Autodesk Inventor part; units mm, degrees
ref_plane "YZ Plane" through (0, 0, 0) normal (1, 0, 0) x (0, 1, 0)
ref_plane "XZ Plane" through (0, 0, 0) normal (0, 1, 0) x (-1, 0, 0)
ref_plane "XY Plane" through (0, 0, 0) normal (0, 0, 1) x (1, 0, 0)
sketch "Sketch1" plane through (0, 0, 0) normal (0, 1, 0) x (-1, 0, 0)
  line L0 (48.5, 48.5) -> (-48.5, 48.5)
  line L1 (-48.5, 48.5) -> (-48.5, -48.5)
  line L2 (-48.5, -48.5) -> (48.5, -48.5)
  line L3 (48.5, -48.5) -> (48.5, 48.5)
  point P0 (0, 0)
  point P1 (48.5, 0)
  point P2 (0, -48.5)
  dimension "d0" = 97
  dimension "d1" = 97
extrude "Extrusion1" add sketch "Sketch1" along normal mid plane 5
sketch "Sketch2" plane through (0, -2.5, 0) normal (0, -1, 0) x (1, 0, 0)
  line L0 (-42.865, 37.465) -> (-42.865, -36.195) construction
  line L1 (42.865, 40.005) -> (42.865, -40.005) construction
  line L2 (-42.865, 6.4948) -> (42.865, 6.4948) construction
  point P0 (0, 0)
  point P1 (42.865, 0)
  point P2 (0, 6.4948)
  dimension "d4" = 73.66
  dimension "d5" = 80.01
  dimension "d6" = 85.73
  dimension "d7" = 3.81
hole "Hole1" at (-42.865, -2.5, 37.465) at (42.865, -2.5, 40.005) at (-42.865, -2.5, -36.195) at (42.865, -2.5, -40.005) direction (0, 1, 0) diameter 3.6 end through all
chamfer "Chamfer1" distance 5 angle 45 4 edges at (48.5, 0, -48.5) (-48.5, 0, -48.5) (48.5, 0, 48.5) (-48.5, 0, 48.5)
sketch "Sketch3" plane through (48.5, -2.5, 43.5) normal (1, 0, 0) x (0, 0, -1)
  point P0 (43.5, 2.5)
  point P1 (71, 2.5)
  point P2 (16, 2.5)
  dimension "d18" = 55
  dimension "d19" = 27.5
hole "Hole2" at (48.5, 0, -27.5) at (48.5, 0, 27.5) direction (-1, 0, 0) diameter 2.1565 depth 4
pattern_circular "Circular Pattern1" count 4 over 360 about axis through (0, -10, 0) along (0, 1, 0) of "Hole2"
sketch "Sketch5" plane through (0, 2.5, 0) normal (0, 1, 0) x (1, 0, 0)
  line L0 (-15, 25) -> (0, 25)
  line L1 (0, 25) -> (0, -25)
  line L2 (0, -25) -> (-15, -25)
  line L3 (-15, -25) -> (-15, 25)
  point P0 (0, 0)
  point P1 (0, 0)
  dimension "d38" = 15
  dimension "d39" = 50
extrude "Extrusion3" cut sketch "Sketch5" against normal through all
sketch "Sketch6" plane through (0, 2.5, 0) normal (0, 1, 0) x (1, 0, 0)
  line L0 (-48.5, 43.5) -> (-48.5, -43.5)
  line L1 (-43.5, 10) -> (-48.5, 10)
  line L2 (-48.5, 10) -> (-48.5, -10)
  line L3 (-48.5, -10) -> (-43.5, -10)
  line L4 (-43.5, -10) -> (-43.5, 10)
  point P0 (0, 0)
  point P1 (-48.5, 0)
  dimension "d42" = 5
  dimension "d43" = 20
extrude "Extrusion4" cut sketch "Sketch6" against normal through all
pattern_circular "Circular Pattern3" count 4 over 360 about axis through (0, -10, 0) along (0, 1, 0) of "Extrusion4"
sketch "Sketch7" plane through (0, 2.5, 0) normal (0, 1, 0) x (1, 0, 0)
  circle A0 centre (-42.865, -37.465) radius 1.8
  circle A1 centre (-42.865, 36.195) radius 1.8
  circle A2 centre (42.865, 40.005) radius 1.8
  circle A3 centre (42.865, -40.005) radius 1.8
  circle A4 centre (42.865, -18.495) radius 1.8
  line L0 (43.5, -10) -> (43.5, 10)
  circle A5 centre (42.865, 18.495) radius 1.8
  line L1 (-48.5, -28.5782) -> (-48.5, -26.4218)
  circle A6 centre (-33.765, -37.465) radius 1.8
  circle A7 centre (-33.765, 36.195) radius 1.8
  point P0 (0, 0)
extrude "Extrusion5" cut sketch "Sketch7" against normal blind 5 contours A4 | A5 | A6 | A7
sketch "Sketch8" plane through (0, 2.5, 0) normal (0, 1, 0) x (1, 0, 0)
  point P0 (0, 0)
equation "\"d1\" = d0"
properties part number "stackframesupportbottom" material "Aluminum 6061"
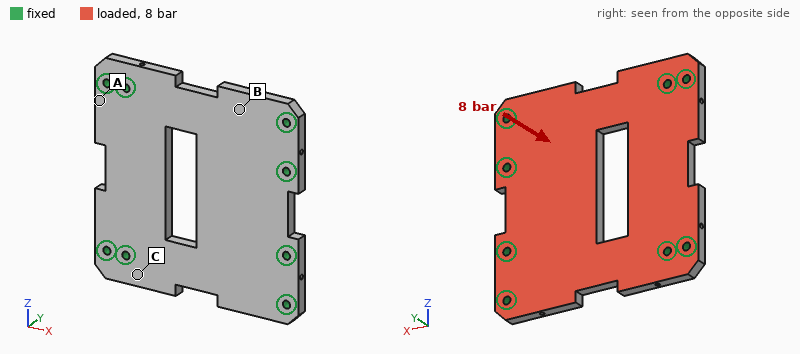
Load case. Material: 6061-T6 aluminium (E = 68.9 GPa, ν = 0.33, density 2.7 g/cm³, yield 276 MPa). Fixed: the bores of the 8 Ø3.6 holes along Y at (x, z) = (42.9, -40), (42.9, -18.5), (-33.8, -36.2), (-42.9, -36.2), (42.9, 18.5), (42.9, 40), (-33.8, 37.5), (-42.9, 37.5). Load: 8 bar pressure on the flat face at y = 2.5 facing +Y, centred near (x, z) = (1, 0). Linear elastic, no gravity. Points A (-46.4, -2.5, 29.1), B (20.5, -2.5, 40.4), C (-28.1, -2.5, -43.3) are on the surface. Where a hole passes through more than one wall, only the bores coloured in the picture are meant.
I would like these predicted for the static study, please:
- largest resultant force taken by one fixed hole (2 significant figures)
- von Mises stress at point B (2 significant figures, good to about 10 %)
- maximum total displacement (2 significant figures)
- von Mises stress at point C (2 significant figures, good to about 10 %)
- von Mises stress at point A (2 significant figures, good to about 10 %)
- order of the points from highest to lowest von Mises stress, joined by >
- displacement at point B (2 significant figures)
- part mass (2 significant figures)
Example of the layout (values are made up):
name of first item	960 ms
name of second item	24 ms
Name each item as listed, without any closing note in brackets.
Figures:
largest resultant force taken by one fixed hole	1.9 kN
von Mises stress at point B	17 MPa
maximum total displacement	0.24 mm
von Mises stress at point C	62 MPa
von Mises stress at point A	43 MPa
order of the points from highest to lowest von Mises stress, joined by >	C > A > B
displacement at point B	0.085 mm
part mass	110 g
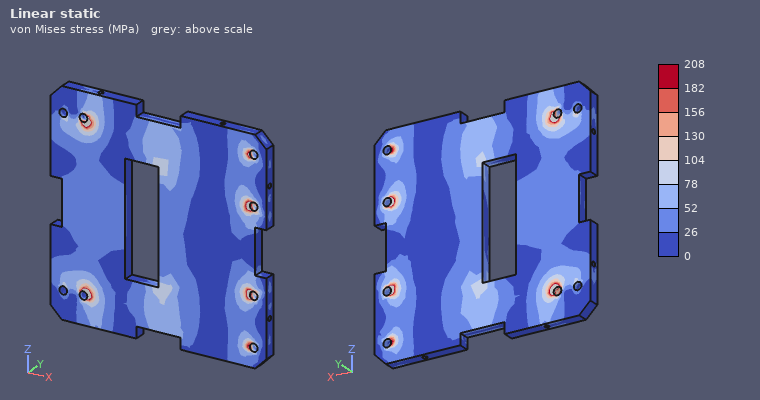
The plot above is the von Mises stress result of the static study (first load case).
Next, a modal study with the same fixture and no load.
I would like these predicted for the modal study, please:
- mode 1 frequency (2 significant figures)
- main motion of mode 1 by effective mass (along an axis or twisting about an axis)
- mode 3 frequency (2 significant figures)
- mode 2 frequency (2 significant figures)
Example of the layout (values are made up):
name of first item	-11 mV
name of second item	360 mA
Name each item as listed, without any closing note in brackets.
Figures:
mode 1 frequency	3400 Hz
main motion of mode 1 by effective mass	along Y
mode 3 frequency	4800 Hz
mode 2 frequency	4800 Hz
